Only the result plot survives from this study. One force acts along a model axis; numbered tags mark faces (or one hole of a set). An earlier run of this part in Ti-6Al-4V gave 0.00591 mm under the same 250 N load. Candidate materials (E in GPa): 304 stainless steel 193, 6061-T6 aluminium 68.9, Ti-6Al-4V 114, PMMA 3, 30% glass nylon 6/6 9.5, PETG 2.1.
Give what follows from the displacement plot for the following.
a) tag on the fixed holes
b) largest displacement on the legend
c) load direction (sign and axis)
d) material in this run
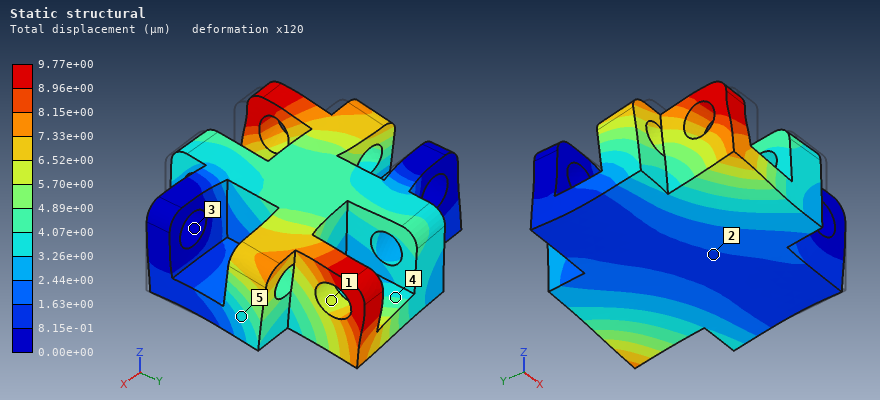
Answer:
3
9.77e+00 µm
+Y
6061-T6 aluminium
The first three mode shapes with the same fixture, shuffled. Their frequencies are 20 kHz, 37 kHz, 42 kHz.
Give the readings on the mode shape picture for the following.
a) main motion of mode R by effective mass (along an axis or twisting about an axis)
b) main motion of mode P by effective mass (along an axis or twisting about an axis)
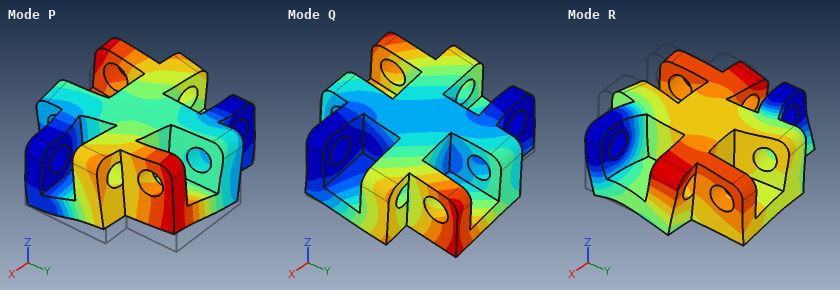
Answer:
along Y
along Z
